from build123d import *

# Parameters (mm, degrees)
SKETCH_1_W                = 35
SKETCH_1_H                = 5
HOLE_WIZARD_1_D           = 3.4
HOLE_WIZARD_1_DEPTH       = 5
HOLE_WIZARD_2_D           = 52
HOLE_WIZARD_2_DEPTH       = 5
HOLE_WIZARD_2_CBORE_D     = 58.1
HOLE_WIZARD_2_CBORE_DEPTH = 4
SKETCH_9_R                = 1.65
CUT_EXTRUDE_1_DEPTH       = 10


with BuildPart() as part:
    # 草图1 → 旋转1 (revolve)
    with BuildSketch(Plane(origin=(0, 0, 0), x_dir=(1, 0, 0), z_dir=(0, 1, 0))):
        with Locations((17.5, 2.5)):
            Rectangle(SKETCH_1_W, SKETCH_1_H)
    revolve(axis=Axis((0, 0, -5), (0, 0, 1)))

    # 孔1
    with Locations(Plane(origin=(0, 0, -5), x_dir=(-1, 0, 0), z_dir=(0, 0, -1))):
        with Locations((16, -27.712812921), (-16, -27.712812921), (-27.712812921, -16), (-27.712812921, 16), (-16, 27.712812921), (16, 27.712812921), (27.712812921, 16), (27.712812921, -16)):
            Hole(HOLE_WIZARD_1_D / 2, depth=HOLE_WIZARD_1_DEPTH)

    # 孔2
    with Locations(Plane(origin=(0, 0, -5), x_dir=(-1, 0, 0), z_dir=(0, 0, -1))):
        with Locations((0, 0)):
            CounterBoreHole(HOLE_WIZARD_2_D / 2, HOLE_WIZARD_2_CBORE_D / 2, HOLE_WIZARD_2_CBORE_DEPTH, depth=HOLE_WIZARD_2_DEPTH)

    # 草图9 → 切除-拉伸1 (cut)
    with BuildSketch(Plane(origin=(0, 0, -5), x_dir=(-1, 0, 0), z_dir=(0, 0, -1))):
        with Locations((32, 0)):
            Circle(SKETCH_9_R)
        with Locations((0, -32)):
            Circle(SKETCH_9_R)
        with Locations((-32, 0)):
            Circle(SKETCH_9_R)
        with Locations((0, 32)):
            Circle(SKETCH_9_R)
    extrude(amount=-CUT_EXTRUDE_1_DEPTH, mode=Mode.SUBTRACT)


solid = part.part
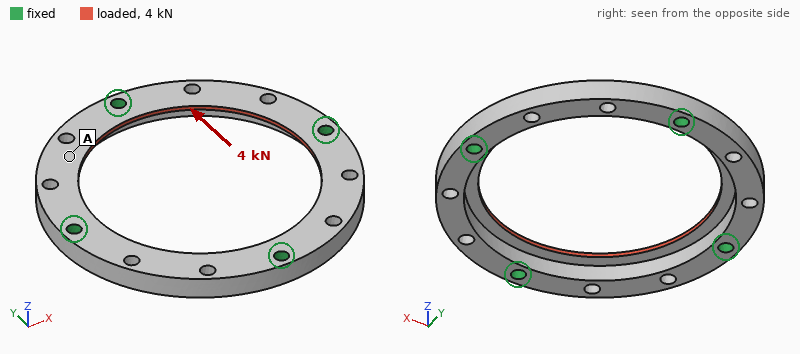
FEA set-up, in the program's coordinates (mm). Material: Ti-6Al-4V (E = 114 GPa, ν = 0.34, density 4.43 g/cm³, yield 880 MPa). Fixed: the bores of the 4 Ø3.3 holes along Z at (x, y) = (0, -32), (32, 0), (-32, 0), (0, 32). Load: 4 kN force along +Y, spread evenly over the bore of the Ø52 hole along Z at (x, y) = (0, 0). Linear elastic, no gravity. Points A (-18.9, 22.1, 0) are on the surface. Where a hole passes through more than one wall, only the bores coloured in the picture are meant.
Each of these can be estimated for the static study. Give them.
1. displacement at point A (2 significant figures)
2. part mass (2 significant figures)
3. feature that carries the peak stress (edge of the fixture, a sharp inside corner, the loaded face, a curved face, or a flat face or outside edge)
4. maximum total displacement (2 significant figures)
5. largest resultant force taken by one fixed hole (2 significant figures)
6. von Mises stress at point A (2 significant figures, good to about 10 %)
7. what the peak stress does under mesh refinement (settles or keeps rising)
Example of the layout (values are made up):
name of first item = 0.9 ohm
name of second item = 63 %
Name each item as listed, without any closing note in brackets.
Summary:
displacement at point A = 12 µm
part mass = 26 g
feature that carries the peak stress = edge of the fixture
maximum total displacement = 15 µm
largest resultant force taken by one fixed hole = 1.4 kN
von Mises stress at point A = 25 MPa
what the peak stress does under mesh refinement = keeps rising
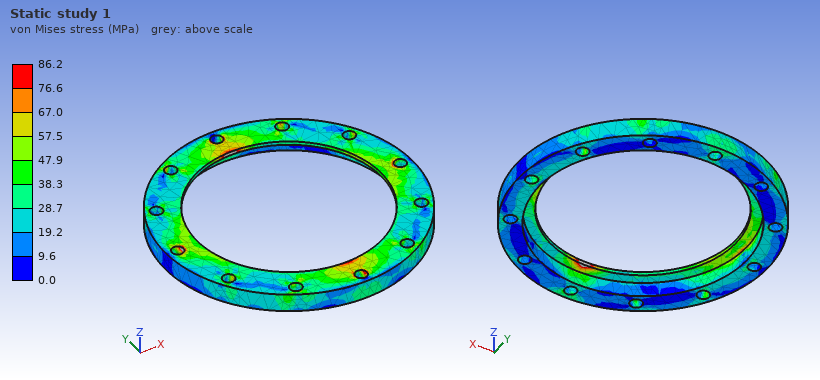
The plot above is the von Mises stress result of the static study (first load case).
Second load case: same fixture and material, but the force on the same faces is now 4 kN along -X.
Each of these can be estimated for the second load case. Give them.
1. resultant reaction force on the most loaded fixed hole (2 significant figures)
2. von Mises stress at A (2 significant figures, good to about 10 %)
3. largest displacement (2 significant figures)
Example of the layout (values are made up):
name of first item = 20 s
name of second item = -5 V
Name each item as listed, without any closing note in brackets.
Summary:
resultant reaction force on the most loaded fixed hole = 1.4 kN
von Mises stress at A = 22 MPa
largest displacement = 15 µm
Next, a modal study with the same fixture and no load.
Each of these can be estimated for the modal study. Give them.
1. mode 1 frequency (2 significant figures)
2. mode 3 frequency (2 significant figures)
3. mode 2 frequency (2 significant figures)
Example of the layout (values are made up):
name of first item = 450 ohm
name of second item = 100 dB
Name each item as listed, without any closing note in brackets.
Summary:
mode 1 frequency = 9800 Hz
mode 3 frequency = 10000 Hz
mode 2 frequency = 10000 Hz
